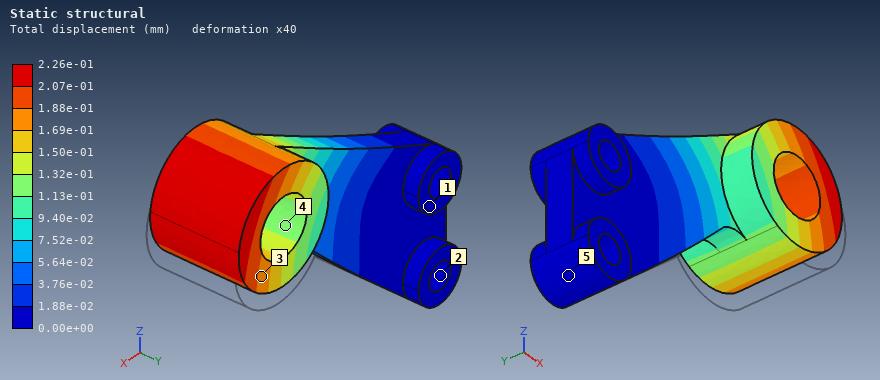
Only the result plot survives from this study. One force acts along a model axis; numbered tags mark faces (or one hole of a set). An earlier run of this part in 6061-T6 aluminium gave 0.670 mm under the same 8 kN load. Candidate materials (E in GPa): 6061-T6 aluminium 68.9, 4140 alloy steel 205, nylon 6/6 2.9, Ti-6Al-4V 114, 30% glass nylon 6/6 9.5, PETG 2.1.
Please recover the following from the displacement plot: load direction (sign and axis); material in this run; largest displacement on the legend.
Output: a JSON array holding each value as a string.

["+Z", "4140 alloy steel", "2.26e-01 mm"]
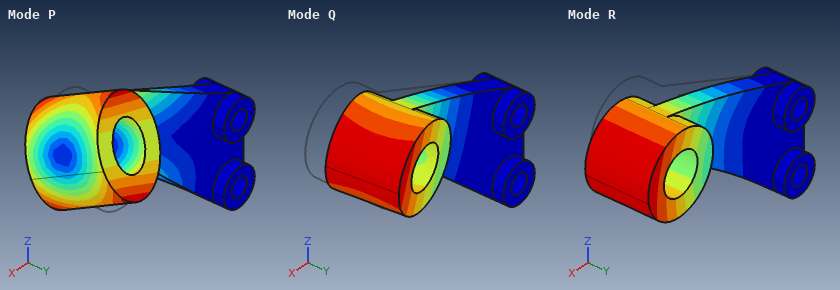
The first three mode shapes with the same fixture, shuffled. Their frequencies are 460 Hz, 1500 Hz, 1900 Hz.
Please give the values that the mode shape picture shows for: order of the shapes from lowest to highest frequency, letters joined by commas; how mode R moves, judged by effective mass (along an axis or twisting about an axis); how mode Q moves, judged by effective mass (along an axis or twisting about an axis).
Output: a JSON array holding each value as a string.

["Q, R, P", "along Z", "along Y"]
